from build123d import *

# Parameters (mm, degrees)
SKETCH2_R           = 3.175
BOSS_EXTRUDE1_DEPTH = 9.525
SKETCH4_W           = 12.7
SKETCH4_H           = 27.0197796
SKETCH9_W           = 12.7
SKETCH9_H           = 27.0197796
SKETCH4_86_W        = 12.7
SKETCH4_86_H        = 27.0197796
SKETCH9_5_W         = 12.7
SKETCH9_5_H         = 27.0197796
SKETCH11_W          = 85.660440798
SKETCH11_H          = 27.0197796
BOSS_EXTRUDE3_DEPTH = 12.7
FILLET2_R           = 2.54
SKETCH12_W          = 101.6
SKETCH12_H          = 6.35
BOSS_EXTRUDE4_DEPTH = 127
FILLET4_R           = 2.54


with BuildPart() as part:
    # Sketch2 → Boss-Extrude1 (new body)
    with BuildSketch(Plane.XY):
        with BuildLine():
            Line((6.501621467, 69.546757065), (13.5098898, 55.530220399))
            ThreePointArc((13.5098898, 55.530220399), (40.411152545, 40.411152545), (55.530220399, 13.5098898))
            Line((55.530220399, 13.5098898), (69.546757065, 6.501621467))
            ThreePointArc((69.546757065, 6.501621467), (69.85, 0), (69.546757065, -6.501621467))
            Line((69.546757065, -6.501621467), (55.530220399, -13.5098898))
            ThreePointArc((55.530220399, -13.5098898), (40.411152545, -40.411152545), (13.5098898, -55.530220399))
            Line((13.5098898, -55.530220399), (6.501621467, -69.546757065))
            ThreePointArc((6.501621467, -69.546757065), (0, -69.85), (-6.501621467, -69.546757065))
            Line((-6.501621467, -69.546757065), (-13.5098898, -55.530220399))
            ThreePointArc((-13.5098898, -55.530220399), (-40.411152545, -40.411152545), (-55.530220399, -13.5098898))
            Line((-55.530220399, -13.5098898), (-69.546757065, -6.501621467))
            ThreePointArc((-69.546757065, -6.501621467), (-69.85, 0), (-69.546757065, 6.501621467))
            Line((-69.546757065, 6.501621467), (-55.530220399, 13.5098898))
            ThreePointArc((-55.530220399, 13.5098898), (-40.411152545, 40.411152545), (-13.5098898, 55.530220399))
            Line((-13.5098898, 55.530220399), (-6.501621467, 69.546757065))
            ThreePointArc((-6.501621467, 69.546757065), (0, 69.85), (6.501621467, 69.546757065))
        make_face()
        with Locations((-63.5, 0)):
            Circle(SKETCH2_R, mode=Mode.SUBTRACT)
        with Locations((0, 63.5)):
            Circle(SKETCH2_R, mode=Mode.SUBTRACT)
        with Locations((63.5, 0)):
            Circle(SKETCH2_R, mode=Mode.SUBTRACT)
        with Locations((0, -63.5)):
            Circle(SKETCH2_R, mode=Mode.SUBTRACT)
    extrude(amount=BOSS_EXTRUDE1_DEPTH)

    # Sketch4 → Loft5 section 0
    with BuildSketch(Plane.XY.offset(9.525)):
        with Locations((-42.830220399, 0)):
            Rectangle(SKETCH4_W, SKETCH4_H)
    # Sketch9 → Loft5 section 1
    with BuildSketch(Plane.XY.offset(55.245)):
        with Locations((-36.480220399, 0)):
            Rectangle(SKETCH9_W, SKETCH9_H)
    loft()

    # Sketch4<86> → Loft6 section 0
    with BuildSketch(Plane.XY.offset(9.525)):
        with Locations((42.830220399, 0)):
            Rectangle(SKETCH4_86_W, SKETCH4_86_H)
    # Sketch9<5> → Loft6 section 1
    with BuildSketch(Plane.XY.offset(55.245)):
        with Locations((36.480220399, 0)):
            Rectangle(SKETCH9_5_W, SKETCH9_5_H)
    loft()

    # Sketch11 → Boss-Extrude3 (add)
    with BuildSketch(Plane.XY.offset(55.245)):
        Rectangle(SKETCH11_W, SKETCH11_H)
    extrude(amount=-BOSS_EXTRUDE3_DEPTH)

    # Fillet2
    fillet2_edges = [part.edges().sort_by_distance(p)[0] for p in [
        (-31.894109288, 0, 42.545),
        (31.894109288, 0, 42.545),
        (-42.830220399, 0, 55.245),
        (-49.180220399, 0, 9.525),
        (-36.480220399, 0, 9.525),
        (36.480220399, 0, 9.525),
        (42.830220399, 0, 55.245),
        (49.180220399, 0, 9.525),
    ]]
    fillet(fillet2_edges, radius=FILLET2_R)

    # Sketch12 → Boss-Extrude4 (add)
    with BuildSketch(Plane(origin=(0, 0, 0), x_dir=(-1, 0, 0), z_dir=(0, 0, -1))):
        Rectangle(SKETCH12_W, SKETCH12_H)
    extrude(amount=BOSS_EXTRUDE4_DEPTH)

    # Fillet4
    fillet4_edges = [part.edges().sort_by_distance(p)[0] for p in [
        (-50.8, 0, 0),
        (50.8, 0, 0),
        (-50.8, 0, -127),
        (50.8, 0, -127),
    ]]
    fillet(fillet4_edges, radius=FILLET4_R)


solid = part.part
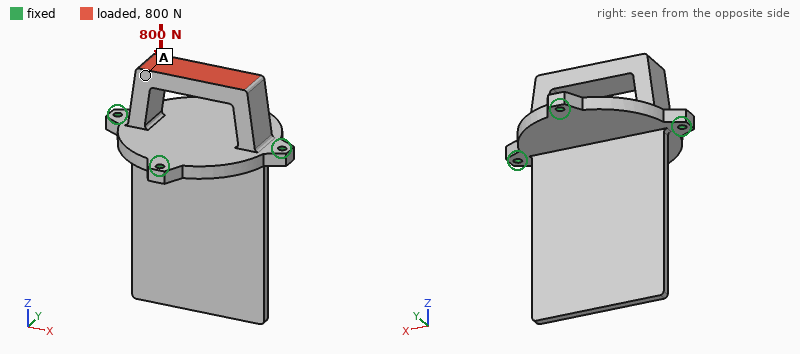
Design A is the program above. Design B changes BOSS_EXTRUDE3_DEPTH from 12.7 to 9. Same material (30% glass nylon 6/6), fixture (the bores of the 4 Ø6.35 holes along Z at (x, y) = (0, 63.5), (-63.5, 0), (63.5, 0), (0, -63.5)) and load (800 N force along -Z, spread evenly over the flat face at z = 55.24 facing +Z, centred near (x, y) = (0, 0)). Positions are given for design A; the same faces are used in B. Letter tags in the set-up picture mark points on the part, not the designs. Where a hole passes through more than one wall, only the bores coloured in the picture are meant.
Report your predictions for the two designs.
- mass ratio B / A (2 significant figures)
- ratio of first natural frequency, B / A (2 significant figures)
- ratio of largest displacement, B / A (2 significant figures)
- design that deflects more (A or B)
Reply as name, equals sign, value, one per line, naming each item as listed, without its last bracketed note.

mass ratio B / A = 0.97
ratio of first natural frequency, B / A = 1.0
ratio of largest displacement, B / A = 1.5
design that deflects more = B
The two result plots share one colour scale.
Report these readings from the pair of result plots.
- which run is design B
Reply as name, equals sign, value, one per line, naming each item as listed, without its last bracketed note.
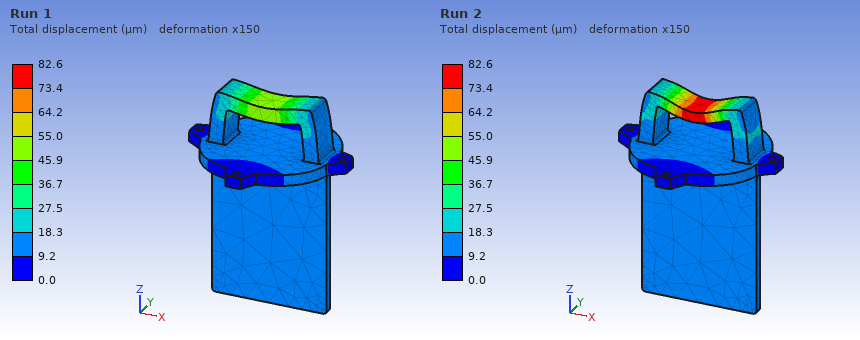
which run is design B = Run 2
